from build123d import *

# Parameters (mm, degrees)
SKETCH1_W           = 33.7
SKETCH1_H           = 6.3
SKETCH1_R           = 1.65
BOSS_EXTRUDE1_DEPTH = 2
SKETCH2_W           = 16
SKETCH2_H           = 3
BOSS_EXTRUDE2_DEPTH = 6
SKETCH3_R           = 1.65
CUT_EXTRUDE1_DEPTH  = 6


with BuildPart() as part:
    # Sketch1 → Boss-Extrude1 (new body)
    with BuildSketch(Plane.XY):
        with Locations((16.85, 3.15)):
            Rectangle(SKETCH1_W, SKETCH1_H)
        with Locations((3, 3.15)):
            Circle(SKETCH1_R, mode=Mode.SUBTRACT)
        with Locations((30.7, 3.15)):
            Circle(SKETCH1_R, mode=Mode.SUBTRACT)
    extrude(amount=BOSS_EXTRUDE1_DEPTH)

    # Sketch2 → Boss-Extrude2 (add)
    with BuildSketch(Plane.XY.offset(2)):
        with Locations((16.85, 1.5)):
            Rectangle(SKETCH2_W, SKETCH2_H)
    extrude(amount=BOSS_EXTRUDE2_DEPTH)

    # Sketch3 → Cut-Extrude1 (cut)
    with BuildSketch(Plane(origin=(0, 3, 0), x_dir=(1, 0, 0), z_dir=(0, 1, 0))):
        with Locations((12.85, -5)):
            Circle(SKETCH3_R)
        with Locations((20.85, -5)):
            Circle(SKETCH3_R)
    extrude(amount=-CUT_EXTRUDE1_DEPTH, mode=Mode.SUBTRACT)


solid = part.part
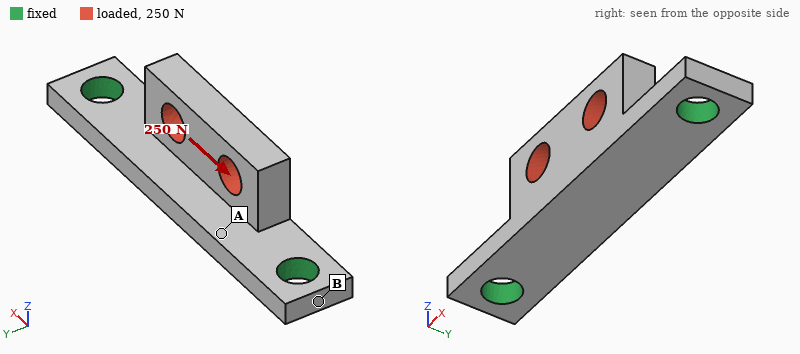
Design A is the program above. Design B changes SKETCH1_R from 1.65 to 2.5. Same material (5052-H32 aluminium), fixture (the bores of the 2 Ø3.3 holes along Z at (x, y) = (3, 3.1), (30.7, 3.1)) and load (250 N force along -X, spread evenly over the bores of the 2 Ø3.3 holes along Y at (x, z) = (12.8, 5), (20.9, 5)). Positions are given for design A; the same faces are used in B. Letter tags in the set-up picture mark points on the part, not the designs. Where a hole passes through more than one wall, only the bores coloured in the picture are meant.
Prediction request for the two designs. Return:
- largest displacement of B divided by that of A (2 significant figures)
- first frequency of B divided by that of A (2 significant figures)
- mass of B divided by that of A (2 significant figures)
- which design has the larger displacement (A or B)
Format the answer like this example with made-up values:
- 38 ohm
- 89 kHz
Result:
- 0.81
- 1.1
- 0.93
- A
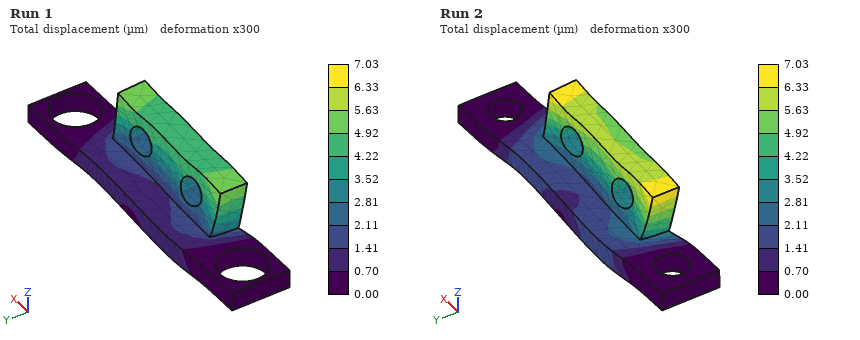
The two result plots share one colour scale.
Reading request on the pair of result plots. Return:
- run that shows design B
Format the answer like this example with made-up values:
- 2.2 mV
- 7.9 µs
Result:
- Run 1
